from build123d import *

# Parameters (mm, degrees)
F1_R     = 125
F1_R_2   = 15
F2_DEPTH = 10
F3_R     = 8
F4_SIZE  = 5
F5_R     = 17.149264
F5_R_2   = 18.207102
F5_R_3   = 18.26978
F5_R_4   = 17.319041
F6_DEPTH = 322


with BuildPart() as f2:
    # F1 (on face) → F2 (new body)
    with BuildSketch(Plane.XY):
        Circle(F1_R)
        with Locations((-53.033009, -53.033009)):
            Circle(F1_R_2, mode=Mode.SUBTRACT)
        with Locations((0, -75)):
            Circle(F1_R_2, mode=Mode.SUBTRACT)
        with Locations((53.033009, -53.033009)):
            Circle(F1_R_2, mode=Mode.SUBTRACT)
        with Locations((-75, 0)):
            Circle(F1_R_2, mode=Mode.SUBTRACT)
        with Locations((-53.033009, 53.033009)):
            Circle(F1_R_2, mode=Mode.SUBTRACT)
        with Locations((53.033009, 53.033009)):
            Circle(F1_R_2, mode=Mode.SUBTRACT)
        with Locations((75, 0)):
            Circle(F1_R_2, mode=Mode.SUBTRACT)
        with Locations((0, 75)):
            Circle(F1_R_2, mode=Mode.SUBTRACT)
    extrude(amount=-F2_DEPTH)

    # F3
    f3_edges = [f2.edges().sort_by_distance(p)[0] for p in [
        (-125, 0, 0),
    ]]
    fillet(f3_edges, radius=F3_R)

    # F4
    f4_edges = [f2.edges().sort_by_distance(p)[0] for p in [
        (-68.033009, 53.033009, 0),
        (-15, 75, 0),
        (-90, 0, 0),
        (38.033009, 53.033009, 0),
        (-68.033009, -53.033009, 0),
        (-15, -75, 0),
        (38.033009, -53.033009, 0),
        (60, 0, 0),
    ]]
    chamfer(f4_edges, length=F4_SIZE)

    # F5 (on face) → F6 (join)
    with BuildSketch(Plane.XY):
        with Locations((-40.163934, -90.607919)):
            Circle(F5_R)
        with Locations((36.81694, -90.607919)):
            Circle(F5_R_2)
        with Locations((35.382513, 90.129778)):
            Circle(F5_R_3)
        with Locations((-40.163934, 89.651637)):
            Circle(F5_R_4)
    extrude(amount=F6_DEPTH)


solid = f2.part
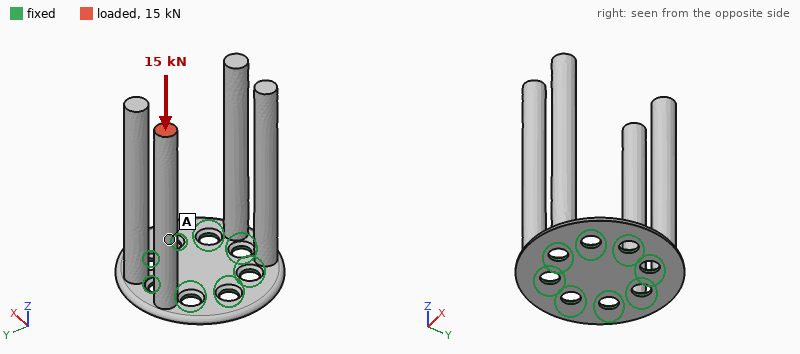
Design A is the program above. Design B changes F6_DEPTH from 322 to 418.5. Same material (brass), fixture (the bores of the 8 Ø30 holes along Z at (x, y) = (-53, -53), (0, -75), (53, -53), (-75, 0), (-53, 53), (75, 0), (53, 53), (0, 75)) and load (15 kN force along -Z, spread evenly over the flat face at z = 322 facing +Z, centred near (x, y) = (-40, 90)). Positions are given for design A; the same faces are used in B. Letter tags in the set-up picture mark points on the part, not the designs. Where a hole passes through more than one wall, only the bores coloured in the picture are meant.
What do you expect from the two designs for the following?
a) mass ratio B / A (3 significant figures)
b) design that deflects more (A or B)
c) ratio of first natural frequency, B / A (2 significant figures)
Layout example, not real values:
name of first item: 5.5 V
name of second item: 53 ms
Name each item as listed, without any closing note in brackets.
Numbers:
mass ratio B / A: 1.23
design that deflects more: B
ratio of first natural frequency, B / A: 0.64
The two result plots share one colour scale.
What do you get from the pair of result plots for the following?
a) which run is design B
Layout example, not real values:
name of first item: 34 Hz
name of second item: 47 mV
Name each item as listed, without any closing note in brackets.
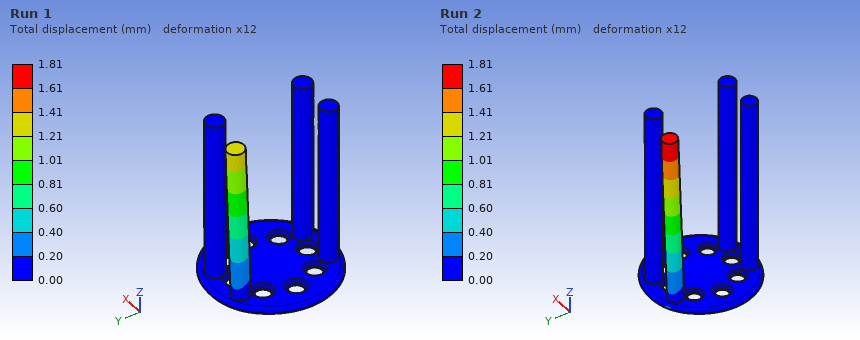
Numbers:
which run is design B: Run 2
